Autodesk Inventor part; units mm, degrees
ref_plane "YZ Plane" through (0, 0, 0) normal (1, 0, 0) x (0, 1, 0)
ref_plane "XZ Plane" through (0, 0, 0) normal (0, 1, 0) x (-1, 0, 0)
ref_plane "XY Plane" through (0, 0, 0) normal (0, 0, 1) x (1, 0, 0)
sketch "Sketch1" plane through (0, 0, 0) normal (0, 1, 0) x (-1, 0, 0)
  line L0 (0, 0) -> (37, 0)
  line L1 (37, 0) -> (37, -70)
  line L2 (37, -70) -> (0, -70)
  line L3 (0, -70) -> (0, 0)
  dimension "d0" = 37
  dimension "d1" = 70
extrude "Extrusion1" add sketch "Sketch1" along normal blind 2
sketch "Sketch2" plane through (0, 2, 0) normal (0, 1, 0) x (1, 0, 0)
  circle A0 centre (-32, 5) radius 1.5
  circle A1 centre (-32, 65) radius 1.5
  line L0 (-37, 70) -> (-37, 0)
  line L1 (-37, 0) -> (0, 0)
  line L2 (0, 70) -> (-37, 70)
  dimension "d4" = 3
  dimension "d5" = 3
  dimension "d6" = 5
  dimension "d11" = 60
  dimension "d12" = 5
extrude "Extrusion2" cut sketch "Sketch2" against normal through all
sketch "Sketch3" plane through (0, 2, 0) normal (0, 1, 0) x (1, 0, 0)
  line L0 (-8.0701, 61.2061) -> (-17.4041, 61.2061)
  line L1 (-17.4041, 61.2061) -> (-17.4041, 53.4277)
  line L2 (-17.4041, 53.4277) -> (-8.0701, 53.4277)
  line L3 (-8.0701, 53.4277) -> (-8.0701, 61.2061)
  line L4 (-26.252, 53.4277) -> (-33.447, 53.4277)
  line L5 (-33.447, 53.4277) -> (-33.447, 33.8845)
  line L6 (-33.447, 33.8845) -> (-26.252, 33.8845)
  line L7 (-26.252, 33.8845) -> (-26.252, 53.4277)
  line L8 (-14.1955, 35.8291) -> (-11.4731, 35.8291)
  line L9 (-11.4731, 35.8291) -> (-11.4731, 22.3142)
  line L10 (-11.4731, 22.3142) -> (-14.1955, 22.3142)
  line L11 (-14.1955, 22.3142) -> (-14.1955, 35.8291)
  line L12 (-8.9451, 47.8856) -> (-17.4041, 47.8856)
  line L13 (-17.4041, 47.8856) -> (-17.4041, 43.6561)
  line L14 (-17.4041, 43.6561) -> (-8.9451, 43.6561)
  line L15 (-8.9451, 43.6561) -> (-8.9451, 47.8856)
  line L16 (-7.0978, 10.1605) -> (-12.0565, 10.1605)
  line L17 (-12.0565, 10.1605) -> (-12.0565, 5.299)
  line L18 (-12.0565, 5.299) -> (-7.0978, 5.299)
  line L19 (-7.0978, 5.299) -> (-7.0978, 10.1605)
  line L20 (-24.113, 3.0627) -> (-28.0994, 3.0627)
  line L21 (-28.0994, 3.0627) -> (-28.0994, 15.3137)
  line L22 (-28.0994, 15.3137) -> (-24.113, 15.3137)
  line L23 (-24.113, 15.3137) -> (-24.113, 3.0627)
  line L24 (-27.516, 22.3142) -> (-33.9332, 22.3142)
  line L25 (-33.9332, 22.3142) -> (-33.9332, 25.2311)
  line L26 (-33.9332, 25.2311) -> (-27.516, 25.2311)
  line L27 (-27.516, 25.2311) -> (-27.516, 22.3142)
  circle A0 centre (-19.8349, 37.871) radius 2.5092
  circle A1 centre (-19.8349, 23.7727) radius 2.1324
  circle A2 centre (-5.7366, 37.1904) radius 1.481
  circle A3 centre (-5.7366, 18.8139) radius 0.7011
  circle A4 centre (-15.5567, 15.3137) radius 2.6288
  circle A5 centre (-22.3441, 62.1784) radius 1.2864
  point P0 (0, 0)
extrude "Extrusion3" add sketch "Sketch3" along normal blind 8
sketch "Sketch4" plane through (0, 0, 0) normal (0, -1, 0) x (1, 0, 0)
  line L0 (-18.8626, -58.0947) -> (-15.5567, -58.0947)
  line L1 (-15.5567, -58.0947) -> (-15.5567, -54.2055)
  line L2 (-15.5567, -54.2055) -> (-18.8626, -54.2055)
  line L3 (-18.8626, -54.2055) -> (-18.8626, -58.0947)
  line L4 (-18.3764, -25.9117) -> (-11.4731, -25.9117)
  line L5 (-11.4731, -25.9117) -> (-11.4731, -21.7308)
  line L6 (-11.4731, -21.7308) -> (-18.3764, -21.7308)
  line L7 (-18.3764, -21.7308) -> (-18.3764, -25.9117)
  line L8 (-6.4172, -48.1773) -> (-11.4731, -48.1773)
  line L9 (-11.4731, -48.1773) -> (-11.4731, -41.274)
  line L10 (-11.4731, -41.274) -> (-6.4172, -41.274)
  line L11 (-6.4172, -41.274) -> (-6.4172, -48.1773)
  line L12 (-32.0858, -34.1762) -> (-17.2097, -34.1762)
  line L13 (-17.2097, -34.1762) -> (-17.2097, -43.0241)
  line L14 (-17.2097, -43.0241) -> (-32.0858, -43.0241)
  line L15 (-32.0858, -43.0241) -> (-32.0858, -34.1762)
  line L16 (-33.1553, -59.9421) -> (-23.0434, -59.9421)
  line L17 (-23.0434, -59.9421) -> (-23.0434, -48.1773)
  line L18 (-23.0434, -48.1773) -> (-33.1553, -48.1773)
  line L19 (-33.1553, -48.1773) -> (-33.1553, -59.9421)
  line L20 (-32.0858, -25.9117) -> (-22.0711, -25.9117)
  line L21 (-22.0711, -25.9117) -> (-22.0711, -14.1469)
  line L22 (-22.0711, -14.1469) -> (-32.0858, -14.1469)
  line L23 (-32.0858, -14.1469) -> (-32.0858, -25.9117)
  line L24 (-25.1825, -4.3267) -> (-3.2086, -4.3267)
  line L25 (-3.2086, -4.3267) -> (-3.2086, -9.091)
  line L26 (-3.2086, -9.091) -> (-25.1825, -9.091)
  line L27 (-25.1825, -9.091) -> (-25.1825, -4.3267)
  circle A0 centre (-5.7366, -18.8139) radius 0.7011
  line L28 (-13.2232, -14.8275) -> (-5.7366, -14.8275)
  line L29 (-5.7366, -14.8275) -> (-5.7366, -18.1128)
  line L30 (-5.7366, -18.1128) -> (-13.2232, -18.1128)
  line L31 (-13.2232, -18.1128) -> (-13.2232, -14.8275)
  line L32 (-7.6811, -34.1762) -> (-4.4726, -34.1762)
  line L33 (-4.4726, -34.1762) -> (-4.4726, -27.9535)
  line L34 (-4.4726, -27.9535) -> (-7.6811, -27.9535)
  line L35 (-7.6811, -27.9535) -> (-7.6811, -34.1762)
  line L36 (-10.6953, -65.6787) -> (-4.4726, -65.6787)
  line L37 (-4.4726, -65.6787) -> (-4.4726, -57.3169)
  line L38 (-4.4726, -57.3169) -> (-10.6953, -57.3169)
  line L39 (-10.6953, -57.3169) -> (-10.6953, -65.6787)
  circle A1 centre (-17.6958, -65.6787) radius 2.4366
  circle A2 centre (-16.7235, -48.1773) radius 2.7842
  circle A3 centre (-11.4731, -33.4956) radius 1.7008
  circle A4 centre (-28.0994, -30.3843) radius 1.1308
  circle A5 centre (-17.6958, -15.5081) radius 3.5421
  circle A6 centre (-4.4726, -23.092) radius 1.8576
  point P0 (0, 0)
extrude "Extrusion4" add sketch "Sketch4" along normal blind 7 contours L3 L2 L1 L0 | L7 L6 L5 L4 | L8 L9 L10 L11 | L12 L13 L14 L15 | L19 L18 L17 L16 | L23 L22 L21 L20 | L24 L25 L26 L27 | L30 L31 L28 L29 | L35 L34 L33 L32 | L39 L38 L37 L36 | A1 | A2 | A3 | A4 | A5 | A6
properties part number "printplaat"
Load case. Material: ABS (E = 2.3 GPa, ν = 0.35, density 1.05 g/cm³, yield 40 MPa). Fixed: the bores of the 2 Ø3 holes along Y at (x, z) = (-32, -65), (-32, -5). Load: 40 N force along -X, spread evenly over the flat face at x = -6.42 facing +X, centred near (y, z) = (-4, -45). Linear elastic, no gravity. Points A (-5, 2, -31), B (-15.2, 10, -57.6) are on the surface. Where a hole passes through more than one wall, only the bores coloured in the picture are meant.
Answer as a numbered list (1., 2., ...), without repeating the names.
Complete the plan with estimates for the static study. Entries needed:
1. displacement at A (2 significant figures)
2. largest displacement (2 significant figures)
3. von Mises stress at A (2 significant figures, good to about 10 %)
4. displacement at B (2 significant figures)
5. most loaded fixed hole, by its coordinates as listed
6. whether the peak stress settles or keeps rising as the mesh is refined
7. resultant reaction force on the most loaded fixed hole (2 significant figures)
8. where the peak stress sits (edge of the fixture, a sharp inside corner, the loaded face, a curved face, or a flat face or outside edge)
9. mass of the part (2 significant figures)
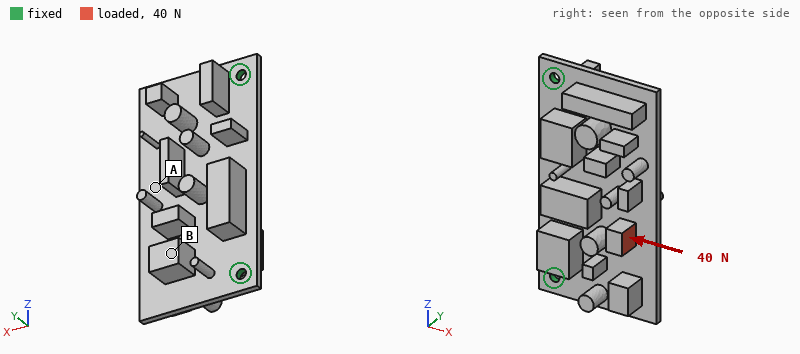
1. 0.52 mm
2. 0.78 mm
3. 1.7 MPa
4. 0.39 mm
5. (-32, -65)
6. keeps rising
7. 28 N
8. edge of the fixture
9. 15 g
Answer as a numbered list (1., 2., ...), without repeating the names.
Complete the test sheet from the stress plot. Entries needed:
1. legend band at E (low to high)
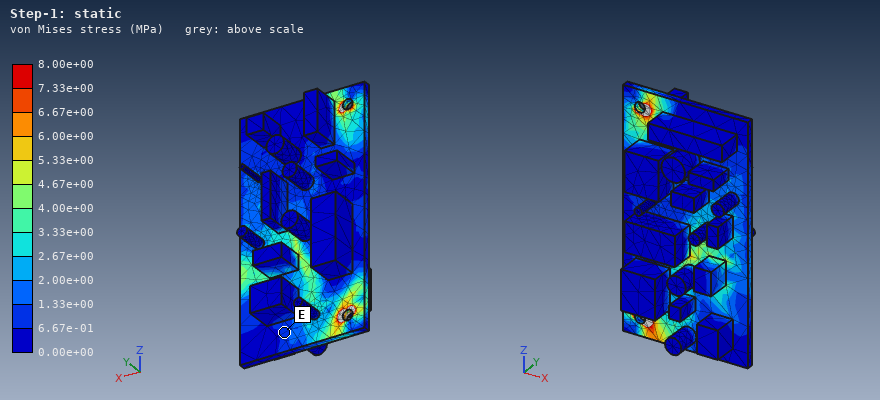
1. 6.67e-01 to 1.33e+00 MPa
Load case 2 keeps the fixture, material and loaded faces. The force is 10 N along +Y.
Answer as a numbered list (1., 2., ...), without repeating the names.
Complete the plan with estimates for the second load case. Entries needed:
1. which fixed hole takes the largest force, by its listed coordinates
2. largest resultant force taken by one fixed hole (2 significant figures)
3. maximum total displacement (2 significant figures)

1. (-32, -65)
2. 6.3 N
3. 0.96 mm
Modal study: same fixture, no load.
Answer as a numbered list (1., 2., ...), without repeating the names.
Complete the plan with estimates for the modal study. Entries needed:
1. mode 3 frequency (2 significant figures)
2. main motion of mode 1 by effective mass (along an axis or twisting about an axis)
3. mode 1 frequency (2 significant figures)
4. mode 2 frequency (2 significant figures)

1. 720 Hz
2. along Y
3. 270 Hz
4. 650 Hz
